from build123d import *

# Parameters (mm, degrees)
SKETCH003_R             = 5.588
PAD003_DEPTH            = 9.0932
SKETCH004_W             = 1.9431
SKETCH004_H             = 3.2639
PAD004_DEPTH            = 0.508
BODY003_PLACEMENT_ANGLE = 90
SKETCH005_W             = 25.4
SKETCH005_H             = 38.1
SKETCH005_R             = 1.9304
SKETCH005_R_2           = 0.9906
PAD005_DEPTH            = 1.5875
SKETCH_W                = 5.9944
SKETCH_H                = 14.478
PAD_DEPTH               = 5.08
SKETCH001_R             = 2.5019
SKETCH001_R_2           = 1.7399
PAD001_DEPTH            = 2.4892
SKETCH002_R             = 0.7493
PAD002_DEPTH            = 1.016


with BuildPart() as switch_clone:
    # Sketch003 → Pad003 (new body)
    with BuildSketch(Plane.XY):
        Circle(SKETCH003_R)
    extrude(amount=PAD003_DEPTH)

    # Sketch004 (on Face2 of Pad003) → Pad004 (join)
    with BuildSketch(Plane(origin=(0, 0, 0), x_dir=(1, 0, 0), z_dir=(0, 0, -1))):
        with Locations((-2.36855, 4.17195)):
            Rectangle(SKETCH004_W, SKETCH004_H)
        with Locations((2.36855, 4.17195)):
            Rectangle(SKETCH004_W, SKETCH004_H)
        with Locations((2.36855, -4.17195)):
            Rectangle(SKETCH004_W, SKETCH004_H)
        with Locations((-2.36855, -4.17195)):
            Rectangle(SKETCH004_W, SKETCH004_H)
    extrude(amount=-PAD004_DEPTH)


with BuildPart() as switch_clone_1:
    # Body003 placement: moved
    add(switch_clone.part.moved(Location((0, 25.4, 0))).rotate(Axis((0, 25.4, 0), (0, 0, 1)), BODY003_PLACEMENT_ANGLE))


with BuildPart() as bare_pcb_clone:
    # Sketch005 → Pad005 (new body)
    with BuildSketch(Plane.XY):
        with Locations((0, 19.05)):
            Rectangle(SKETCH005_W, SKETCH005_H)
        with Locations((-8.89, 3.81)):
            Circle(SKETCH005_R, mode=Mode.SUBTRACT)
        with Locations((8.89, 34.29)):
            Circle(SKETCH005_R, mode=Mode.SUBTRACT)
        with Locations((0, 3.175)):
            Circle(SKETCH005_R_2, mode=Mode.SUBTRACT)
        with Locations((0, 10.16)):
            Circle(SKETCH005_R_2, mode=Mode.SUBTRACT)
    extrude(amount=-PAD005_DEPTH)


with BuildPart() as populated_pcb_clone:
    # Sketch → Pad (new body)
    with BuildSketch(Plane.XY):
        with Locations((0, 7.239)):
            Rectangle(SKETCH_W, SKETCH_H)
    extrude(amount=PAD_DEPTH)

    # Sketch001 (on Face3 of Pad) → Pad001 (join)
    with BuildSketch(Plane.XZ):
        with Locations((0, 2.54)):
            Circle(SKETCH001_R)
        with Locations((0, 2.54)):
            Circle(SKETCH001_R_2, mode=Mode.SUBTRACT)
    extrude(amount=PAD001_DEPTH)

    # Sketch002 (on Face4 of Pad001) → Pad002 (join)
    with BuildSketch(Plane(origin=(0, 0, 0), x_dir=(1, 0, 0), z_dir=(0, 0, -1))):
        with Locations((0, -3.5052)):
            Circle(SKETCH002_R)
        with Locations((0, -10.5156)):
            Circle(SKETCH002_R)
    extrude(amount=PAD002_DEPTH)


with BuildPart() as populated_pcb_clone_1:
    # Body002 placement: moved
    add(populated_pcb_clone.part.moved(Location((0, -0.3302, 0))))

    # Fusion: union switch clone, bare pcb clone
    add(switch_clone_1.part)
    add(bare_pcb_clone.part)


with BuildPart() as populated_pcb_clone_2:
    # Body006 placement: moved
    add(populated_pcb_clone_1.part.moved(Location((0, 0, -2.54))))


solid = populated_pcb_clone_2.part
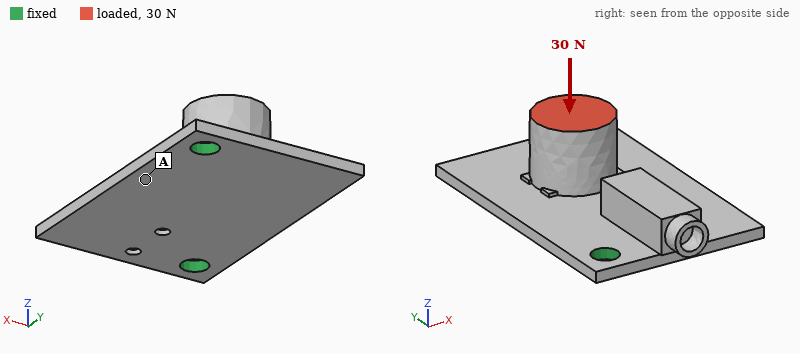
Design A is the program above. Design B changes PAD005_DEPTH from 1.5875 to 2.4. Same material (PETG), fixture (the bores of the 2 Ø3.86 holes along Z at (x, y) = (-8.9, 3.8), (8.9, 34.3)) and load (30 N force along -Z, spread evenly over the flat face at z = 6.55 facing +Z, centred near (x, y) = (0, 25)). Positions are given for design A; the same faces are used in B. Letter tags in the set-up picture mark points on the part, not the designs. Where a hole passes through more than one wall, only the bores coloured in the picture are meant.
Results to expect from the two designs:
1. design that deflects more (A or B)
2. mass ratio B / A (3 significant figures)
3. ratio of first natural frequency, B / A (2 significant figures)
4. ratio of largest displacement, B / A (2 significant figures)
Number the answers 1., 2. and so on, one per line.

1. A
2. 1.27
3. 1.5
4. 0.36
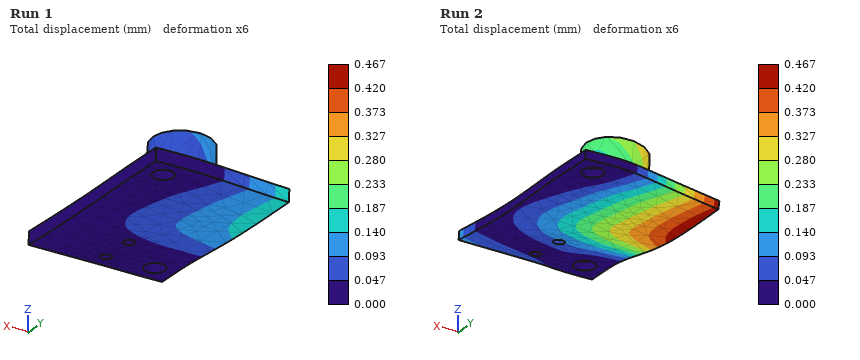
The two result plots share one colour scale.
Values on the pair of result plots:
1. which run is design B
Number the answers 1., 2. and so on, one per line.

1. Run 1
